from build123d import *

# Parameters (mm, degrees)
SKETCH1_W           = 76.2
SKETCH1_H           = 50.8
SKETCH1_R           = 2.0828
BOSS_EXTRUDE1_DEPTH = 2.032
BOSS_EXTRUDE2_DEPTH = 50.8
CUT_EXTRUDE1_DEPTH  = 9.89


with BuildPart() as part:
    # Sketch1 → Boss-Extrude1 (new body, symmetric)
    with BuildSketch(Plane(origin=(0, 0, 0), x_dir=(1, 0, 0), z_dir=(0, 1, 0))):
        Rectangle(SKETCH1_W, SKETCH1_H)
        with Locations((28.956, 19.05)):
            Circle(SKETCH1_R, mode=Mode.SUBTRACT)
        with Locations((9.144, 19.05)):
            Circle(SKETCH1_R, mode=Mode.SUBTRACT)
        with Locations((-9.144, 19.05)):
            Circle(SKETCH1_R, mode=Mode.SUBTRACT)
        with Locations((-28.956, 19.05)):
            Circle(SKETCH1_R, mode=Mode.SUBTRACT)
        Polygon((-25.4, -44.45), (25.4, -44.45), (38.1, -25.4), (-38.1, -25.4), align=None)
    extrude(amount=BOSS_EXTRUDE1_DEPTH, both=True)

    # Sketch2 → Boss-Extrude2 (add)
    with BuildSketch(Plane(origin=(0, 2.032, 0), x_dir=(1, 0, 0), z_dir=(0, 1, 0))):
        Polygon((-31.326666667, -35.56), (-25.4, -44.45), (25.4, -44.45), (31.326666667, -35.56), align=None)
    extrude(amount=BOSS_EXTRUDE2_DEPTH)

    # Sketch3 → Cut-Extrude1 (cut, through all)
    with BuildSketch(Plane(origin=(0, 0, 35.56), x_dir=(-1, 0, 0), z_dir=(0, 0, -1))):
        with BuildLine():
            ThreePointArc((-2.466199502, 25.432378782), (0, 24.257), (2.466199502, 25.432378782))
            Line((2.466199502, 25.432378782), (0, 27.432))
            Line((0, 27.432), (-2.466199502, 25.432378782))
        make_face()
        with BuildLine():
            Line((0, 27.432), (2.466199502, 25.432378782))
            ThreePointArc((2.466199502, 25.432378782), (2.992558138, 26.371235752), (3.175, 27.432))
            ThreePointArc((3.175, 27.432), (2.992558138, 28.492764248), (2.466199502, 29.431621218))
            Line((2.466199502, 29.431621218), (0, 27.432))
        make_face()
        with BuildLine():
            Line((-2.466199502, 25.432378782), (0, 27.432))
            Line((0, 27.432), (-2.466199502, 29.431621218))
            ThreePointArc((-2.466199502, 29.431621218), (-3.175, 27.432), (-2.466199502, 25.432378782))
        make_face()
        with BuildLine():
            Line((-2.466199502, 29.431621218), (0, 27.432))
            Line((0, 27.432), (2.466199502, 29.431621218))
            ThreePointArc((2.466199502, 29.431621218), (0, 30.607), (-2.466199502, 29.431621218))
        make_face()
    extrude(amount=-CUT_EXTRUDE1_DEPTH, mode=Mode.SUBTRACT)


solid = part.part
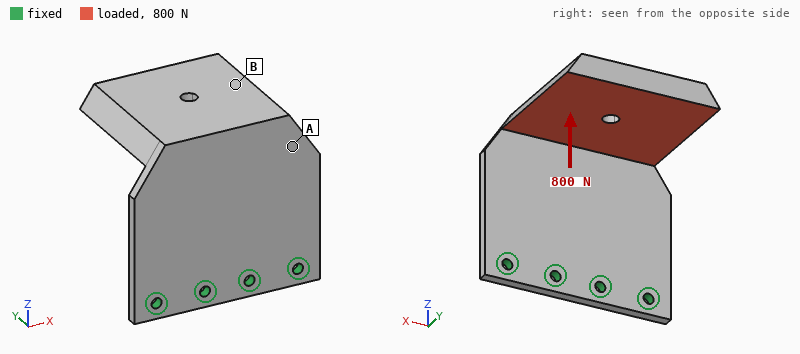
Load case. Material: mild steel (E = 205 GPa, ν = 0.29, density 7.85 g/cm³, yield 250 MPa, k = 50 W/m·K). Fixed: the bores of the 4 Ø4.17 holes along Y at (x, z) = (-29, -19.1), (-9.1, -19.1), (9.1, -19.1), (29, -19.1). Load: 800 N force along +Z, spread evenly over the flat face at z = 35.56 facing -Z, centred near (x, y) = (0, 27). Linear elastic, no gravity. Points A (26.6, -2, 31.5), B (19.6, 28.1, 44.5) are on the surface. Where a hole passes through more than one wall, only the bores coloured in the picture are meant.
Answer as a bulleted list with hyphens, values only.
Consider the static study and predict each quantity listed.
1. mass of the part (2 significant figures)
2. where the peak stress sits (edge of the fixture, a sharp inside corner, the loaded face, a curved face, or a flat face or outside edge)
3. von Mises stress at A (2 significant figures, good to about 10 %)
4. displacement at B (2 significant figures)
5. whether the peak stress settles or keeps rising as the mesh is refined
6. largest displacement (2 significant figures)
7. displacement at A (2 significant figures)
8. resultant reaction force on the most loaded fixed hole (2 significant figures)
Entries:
- 360 g
- edge of the fixture
- 110 MPa
- 0.63 mm
- keeps rising
- 0.90 mm
- 0.31 mm
- 210 N
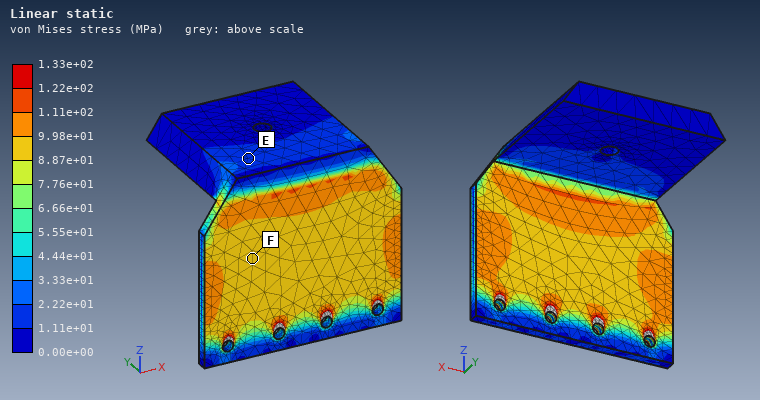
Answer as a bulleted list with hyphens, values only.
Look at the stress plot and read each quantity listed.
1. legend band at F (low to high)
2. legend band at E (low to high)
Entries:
- 8.87e+01 to 9.98e+01 MPa
- 1.11e+01 to 2.22e+01 MPa
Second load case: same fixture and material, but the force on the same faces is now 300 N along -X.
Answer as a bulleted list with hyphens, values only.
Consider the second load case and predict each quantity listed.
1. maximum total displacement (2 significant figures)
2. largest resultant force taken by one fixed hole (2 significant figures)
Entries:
- 0.11 mm
- 290 N
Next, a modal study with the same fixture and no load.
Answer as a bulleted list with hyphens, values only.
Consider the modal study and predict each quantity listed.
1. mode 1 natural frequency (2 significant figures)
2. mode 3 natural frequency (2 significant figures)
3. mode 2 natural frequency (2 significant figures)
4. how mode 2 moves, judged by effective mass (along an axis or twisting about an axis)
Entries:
- 300 Hz
- 1100 Hz
- 650 Hz
- along X
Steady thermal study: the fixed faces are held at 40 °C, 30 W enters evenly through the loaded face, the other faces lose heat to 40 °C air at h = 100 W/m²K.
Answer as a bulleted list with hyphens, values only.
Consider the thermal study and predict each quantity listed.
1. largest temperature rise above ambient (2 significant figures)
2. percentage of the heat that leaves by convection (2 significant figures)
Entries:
- 40 K
- 87 %
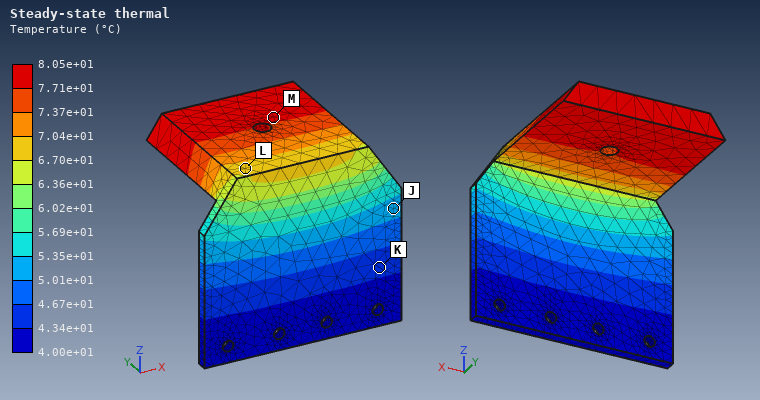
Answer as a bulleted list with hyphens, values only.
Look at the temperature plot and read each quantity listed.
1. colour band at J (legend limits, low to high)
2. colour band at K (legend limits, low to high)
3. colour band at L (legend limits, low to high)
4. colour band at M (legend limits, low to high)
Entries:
- 5.01e+01 to 5.35e+01 °C
- 4.34e+01 to 4.67e+01 °C
- 6.70e+01 to 7.04e+01 °C
- 7.71e+01 to 8.05e+01 °C
